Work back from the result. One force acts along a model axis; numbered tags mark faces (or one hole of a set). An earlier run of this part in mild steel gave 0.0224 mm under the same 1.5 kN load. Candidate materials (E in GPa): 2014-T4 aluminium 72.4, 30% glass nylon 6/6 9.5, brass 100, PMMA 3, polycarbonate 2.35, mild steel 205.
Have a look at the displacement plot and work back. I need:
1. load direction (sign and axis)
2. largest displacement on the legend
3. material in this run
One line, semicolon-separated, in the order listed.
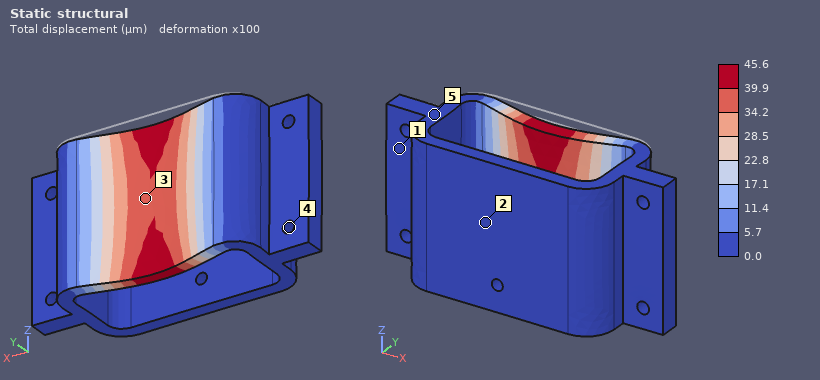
-Y; 45.6 µm; brass
